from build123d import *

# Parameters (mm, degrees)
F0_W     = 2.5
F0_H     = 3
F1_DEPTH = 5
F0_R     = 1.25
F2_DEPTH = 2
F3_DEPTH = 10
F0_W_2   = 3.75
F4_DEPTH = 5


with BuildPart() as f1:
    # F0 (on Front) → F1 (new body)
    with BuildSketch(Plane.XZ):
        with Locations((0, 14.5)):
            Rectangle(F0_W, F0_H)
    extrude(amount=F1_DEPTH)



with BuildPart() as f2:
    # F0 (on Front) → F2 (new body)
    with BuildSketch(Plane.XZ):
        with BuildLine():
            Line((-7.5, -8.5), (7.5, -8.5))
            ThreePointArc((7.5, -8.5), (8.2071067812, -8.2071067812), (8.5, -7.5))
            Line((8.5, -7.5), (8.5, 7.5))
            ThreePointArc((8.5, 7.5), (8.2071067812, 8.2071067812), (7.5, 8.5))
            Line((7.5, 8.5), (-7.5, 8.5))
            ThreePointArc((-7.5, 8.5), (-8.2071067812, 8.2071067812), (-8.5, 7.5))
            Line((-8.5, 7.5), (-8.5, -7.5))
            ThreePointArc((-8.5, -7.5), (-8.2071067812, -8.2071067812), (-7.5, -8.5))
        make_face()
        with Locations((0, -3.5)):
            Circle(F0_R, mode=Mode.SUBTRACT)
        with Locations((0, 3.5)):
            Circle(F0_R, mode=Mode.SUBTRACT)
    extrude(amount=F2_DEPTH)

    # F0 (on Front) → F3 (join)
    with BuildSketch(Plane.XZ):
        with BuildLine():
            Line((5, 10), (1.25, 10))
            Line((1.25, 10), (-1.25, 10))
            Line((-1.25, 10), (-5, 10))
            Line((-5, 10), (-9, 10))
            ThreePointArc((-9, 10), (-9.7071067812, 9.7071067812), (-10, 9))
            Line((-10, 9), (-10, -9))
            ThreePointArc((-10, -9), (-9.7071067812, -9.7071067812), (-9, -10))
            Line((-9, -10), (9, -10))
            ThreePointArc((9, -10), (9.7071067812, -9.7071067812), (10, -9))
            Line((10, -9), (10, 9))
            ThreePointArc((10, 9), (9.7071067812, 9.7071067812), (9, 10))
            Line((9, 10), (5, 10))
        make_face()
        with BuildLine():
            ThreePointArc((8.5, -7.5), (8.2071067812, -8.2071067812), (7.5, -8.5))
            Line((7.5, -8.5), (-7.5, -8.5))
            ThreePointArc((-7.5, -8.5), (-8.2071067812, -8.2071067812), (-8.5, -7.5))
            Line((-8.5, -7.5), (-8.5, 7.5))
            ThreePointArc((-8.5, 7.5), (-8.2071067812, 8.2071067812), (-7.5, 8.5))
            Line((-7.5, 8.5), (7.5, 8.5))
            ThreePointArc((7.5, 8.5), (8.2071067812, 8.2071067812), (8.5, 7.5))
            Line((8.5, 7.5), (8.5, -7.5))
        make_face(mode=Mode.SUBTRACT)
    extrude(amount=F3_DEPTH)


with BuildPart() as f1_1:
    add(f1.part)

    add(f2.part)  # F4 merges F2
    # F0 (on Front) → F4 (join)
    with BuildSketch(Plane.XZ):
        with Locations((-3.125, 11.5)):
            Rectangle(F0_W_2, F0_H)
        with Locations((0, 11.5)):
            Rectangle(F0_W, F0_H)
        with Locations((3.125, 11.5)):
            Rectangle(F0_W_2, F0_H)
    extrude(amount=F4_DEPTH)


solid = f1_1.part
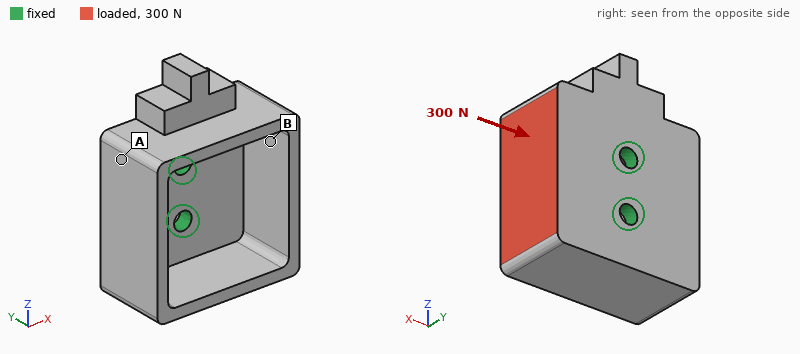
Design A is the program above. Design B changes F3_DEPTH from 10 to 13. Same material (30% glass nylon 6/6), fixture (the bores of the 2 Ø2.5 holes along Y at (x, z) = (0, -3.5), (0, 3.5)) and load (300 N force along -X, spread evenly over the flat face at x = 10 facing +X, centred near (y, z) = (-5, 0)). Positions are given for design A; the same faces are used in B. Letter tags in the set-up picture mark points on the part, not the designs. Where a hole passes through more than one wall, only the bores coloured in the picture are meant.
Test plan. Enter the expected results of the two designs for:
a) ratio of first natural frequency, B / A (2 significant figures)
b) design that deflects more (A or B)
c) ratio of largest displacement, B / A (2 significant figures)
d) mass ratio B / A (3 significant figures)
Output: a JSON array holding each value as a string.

["0.80", "B", "1.3", "1.18"]
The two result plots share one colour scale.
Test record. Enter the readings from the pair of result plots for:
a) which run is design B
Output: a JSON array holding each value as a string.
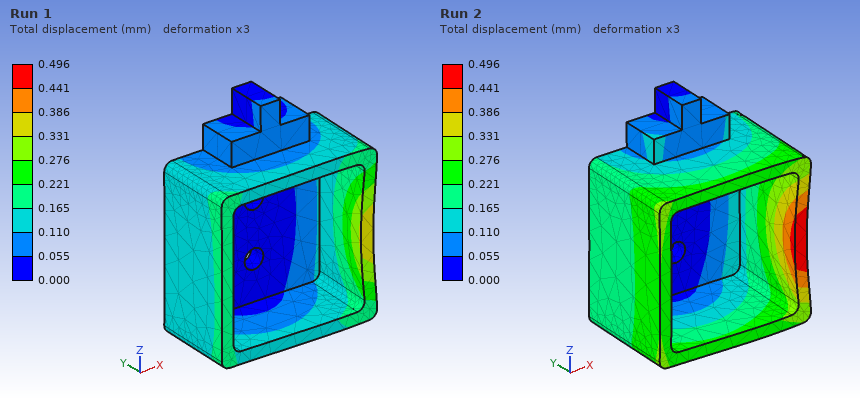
["Run 2"]
